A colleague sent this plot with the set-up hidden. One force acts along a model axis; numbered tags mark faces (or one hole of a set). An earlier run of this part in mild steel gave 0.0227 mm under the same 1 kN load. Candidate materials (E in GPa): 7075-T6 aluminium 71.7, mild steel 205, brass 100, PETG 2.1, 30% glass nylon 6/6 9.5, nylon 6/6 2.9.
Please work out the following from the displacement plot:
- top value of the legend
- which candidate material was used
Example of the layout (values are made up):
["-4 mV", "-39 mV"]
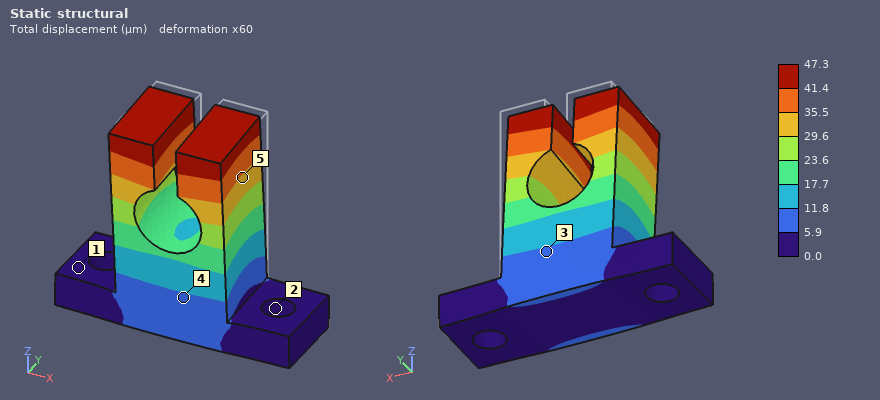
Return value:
["47.3 µm", "brass"]
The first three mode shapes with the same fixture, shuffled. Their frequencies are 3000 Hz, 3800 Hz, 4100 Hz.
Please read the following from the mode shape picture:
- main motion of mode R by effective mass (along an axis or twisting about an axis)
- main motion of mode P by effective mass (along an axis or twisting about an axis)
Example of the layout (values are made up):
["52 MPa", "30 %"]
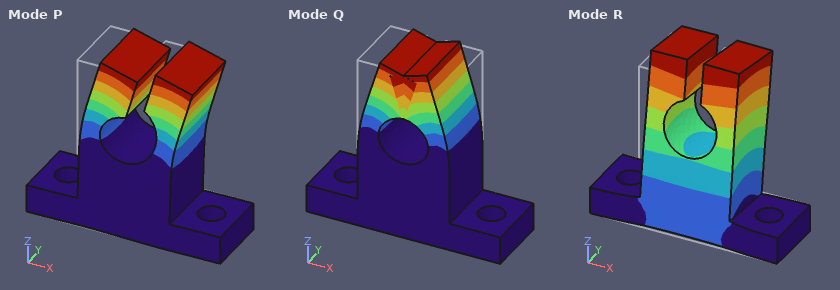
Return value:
["along Y", "along X"]
